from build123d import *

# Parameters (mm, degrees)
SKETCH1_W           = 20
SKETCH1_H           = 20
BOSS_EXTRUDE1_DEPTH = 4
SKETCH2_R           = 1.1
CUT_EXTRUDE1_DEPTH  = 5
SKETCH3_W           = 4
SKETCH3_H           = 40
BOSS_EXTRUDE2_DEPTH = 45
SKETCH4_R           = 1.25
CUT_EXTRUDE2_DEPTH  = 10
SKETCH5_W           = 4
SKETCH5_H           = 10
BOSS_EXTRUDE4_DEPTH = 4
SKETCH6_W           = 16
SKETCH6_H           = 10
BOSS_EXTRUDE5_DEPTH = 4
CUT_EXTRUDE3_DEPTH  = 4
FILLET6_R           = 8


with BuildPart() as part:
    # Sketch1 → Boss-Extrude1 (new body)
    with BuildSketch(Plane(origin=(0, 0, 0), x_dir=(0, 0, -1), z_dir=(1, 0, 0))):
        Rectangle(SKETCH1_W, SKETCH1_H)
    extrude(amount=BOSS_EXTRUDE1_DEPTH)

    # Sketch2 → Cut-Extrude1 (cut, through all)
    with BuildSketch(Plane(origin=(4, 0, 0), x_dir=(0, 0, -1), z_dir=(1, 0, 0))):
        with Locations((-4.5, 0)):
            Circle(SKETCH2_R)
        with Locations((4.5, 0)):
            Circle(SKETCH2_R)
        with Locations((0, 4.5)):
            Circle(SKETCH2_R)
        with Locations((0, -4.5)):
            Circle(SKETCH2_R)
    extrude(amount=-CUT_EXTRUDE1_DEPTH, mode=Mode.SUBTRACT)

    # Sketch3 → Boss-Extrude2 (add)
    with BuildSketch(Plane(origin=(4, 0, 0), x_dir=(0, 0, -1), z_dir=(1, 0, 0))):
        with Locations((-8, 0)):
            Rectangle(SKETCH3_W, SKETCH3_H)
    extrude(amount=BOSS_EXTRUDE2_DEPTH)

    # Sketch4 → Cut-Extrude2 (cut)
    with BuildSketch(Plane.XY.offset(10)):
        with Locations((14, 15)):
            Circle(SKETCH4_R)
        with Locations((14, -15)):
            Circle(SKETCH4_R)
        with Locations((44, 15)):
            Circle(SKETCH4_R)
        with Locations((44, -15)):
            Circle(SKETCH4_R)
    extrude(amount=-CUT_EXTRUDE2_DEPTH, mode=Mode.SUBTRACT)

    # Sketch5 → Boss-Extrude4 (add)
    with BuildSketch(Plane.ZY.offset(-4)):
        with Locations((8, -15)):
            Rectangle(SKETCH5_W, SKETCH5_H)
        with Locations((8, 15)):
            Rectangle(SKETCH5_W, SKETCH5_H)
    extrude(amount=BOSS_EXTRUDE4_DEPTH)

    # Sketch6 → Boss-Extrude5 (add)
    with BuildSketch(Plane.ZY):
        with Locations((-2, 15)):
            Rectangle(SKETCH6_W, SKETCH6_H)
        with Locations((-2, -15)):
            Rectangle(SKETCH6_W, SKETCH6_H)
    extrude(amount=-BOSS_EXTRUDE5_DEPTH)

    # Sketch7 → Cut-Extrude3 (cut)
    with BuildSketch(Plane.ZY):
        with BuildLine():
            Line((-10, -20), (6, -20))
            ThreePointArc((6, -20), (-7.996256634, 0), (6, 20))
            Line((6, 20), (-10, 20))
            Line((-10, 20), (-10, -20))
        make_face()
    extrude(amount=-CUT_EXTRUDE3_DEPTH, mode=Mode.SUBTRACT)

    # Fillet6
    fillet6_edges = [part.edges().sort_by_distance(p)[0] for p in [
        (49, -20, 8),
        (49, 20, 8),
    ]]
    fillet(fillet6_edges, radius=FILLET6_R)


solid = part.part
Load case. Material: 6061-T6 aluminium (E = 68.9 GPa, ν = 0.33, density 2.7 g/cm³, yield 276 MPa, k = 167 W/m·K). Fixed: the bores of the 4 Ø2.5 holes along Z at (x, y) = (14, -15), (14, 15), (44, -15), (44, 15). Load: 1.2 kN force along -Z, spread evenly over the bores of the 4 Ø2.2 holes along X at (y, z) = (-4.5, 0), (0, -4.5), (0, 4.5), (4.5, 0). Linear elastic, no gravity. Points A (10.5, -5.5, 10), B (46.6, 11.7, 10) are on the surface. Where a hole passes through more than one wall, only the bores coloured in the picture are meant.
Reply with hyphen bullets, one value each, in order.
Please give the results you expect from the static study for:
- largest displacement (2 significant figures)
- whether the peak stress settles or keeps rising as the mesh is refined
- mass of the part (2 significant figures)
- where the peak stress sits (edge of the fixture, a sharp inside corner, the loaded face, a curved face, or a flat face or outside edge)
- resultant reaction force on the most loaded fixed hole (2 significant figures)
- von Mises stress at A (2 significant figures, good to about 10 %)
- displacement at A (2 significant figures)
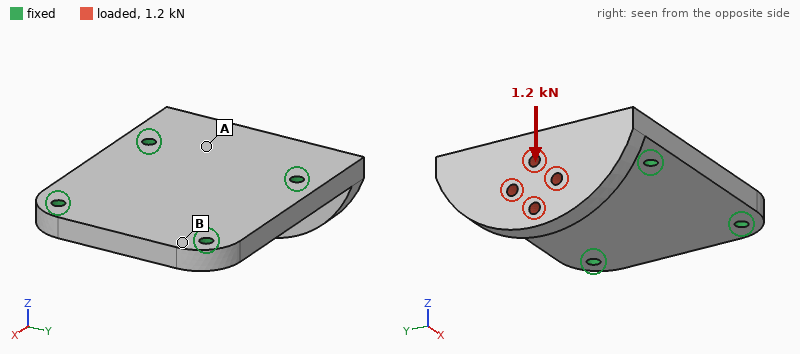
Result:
- 0.15 mm
- keeps rising
- 25 g
- edge of the fixture
- 680 N
- 57 MPa
- 0.024 mm
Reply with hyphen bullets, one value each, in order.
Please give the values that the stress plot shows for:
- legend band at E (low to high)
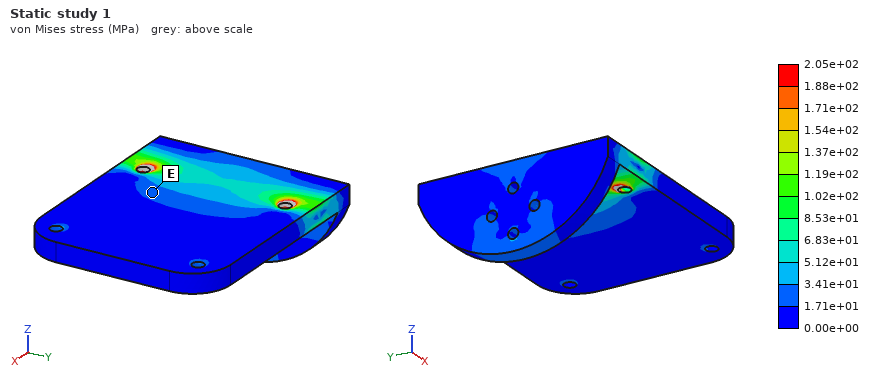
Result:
- 1.71e+01 to 3.41e+01 MPa
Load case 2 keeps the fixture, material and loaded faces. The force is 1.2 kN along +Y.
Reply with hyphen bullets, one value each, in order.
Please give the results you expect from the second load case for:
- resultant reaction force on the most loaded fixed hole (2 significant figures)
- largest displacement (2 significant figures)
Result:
- 790 N
- 32 µm
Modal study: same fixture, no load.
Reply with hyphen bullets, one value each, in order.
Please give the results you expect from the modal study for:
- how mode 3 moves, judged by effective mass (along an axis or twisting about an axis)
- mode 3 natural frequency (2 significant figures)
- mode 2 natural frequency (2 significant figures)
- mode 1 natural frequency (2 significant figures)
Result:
- along Z
- 15 kHz
- 12 kHz
- 6200 Hz
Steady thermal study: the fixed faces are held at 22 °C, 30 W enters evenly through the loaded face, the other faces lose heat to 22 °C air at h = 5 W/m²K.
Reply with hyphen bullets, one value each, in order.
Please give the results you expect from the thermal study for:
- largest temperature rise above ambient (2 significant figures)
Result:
- 34 K
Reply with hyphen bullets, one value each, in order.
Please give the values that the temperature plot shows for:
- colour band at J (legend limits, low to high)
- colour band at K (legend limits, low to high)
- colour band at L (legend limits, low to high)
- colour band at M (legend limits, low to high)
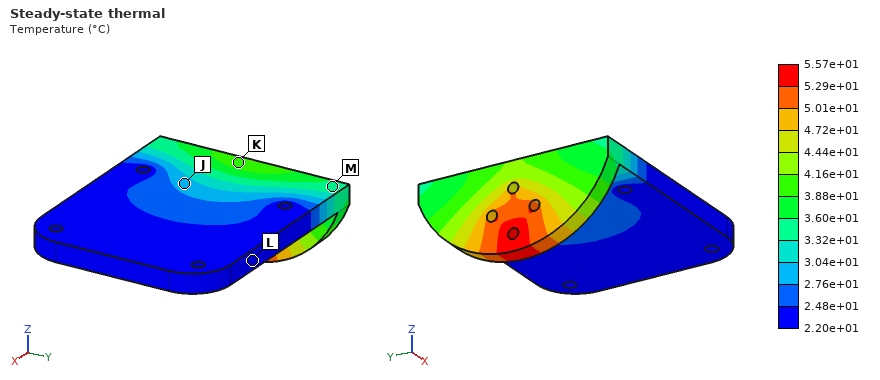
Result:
- 2.76e+01 to 3.04e+01 °C
- 3.88e+01 to 4.16e+01 °C
- 2.20e+01 to 2.48e+01 °C
- 3.32e+01 to 3.60e+01 °C
